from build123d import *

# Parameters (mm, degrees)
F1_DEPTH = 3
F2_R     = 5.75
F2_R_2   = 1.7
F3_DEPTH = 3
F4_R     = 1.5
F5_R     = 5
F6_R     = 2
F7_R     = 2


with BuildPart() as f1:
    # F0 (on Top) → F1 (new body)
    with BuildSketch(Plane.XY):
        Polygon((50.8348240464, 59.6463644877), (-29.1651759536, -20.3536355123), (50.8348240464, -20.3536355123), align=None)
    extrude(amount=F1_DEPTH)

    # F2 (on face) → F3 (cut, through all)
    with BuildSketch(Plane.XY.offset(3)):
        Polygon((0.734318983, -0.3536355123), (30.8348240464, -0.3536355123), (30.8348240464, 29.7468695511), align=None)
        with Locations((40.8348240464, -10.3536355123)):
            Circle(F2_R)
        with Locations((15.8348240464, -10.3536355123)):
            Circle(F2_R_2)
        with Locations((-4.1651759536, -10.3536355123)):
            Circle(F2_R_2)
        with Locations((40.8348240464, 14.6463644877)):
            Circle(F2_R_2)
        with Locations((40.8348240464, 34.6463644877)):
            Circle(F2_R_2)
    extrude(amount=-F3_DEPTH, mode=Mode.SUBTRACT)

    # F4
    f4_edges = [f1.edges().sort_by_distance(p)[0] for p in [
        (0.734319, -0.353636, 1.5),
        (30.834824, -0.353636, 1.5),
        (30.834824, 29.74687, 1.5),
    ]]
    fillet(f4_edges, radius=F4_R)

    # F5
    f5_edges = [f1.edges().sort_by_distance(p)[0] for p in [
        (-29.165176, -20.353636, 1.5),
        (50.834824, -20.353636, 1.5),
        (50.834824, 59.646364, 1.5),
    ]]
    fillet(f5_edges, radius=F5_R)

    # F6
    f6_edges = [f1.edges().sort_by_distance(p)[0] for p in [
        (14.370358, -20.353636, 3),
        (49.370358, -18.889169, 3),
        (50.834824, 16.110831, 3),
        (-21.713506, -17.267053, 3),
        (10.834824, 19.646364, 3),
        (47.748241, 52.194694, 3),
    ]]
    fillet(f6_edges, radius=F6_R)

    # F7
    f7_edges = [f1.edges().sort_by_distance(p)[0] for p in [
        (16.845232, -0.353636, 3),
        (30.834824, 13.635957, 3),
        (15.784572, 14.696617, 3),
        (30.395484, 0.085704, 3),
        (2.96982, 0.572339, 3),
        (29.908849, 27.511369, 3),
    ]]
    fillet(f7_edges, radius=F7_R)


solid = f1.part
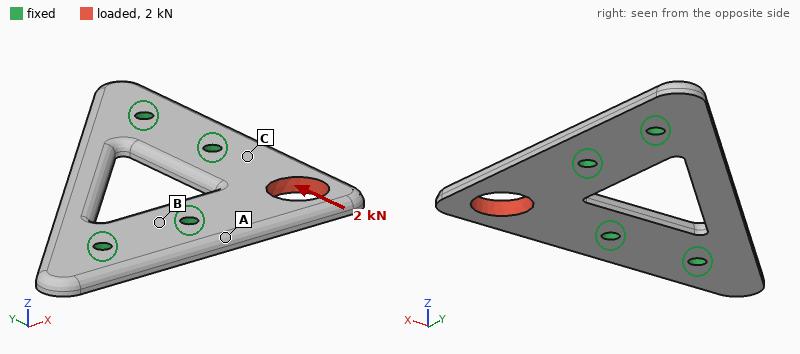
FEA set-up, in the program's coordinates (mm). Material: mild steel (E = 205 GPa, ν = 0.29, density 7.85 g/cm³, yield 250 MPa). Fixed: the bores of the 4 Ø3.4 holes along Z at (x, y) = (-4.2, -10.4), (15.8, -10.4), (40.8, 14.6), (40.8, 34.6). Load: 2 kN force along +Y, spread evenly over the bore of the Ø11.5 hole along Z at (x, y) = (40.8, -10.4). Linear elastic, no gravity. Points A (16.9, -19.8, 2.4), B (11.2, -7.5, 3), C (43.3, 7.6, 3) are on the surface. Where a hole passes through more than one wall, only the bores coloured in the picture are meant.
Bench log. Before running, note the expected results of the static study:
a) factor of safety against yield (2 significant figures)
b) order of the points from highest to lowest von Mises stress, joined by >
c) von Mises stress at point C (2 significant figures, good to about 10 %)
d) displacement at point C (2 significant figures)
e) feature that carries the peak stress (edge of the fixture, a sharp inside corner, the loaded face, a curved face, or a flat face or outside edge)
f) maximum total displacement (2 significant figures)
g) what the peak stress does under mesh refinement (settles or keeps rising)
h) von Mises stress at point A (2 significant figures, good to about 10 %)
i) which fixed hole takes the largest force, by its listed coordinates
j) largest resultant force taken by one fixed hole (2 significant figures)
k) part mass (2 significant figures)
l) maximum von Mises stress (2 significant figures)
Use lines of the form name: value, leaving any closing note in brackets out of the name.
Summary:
factor of safety against yield: 2.5
order of the points from highest to lowest von Mises stress, joined by >: C > A > B
von Mises stress at point C: 38 MPa
displacement at point C: 1.5 µm
feature that carries the peak stress: the loaded face
maximum total displacement: 9.0 µm
what the peak stress does under mesh refinement: settles
von Mises stress at point A: 21 MPa
which fixed hole takes the largest force, by its listed coordinates: (40.8, 14.6)
largest resultant force taken by one fixed hole: 1.4 kN
part mass: 58 g
maximum von Mises stress: 100 MPa
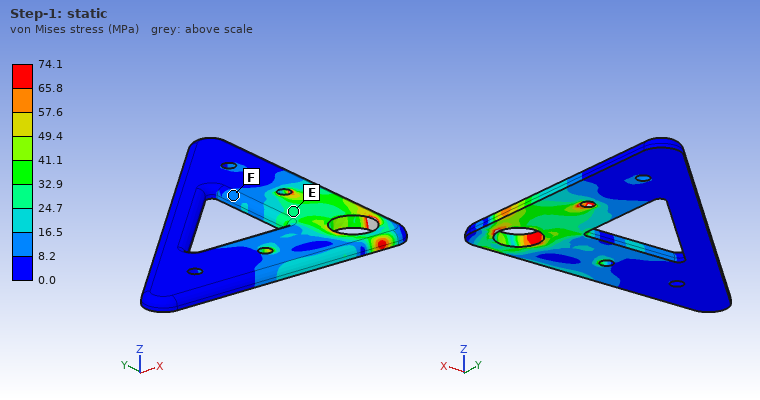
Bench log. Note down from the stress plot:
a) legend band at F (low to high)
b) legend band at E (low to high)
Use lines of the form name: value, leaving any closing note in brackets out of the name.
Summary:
legend band at F: 8.2 to 16.5 MPa
legend band at E: 24.7 to 32.9 MPa
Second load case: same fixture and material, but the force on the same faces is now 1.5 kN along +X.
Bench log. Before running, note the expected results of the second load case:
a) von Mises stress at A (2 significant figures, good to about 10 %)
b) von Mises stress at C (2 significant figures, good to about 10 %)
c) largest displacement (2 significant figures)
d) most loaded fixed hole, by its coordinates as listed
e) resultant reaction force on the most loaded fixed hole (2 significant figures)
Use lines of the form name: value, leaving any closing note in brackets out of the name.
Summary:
von Mises stress at A: 15 MPa
von Mises stress at C: 5.6 MPa
largest displacement: 6.7 µm
most loaded fixed hole, by its coordinates as listed: (15.8, -10.4)
resultant reaction force on the most loaded fixed hole: 1.1 kN
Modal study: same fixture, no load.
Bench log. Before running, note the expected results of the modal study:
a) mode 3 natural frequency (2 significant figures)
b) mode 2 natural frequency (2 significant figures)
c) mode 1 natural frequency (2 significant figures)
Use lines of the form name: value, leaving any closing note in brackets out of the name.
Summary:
mode 3 natural frequency: 9800 Hz
mode 2 natural frequency: 4900 Hz
mode 1 natural frequency: 4200 Hz
